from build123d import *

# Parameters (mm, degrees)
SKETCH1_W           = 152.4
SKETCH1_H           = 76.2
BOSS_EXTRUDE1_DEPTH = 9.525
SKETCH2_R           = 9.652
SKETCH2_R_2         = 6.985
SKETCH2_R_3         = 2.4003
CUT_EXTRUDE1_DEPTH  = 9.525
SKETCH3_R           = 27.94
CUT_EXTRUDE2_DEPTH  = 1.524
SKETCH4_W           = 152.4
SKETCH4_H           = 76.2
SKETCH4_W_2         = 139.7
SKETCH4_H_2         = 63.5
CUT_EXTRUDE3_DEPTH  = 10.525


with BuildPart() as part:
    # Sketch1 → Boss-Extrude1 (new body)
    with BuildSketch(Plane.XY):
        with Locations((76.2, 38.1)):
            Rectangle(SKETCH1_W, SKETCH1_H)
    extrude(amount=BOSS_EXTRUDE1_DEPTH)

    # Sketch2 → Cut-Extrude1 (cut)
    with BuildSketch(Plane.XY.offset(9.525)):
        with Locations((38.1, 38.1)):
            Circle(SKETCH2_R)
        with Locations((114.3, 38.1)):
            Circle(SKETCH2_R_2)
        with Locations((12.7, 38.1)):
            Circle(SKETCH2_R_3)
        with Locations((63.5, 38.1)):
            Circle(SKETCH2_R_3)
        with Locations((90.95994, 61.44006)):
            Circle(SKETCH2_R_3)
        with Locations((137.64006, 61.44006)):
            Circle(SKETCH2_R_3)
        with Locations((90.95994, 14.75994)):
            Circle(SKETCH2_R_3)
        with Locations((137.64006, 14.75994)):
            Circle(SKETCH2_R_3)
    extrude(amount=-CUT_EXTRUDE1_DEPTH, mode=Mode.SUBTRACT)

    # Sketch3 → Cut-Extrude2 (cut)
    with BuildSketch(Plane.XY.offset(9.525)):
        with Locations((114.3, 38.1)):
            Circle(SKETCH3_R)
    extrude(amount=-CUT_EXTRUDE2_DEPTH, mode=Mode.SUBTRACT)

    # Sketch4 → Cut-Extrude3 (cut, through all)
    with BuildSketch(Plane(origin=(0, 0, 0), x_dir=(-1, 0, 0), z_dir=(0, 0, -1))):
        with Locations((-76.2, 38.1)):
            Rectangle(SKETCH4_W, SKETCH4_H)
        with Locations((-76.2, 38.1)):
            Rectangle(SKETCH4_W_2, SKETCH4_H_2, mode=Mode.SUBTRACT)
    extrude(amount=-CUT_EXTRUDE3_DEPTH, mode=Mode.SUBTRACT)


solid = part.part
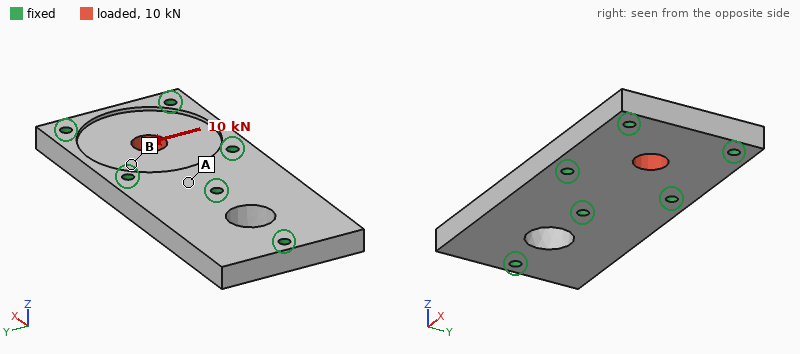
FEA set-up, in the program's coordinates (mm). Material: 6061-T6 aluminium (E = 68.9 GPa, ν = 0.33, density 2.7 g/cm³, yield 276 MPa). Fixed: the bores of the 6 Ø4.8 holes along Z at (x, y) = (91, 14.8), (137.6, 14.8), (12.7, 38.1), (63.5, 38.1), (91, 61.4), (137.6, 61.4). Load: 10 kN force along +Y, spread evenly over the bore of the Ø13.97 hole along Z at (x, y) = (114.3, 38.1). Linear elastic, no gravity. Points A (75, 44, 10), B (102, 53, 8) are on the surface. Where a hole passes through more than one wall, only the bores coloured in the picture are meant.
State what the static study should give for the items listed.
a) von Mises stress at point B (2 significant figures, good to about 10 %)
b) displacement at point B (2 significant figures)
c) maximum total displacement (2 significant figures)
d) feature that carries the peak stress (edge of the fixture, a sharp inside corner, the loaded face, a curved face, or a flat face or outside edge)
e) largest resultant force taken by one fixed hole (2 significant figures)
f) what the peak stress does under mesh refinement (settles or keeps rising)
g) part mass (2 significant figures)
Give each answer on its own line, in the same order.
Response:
22 MPa
5.6 µm
12 µm
edge of the fixture
2.7 kN
keeps rising
200 g
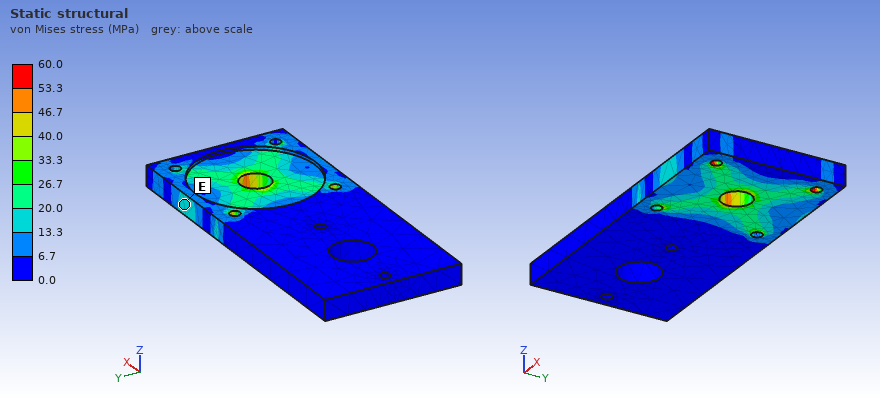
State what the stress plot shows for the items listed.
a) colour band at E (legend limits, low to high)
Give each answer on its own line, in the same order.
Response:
13.3 to 20.0 MPa
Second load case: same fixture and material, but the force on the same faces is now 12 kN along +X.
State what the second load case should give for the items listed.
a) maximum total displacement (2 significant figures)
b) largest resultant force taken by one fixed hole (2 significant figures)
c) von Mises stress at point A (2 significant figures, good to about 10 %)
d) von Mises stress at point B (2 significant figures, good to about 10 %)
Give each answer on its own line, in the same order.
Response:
14 µm
2.8 kN
7.8 MPa
22 MPa
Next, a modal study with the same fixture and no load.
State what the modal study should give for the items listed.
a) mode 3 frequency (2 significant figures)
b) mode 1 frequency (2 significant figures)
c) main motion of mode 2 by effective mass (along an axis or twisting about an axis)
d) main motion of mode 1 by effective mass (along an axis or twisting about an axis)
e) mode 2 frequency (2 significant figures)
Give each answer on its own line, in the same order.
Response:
12 kHz
5800 Hz
along Z
twisting about X
7000 Hz
